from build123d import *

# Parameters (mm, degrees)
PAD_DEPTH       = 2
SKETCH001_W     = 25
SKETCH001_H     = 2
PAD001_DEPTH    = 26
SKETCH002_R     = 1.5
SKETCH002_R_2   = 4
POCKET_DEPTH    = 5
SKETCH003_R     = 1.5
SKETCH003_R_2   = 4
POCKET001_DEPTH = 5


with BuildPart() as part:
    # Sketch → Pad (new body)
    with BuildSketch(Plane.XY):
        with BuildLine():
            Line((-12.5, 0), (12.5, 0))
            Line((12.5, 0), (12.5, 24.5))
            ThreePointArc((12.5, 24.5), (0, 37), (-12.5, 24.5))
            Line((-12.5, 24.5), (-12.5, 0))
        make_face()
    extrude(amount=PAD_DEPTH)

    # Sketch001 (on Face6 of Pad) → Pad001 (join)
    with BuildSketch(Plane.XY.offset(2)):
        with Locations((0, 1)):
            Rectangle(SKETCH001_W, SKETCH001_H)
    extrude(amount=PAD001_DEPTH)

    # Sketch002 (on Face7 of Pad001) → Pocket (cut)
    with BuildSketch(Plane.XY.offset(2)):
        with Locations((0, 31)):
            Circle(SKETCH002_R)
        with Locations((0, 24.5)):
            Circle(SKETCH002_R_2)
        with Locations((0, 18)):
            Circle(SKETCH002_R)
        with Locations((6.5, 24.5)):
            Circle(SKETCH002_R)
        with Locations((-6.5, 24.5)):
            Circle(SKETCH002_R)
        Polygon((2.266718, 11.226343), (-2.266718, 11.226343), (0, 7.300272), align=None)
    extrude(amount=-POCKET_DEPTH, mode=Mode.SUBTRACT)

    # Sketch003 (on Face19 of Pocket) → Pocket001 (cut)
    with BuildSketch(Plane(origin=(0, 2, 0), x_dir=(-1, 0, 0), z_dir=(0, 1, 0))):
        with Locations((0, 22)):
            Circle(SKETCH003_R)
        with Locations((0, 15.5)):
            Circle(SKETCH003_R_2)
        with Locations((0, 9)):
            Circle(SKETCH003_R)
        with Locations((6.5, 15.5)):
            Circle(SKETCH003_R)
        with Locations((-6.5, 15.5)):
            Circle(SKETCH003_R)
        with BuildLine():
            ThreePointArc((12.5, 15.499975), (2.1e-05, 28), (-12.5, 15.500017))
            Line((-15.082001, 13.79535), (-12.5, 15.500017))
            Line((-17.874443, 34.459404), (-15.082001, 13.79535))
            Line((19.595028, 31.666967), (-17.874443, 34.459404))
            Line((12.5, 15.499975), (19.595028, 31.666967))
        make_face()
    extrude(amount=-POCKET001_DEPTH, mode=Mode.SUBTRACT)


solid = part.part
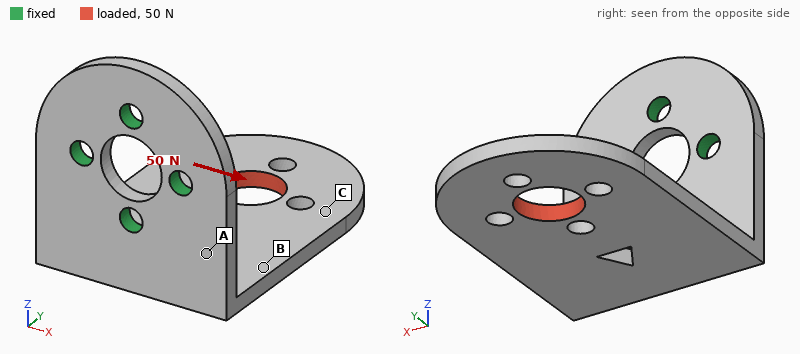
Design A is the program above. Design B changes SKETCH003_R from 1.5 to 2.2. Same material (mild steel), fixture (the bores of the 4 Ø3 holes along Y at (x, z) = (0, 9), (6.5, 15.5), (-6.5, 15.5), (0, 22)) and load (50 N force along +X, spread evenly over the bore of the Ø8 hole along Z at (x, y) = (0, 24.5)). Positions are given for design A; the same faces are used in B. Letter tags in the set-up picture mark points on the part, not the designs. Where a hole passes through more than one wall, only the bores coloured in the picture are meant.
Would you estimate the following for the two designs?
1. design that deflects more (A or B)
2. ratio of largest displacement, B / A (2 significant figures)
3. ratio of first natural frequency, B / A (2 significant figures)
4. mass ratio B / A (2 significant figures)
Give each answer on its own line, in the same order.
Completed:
A
0.83
1.0
0.97
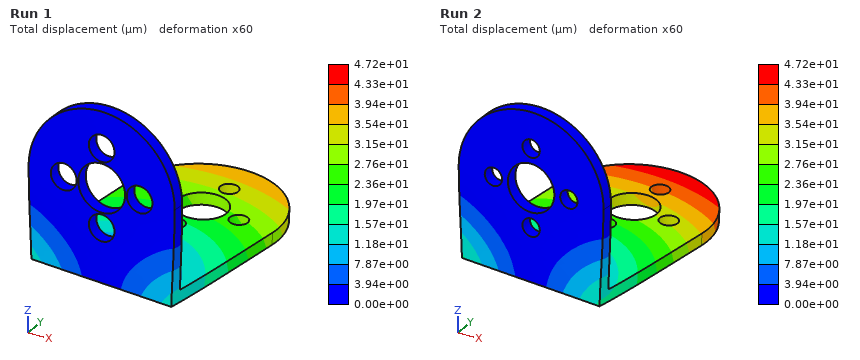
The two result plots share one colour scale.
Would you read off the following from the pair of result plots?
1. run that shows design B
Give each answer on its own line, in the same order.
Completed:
Run 1
